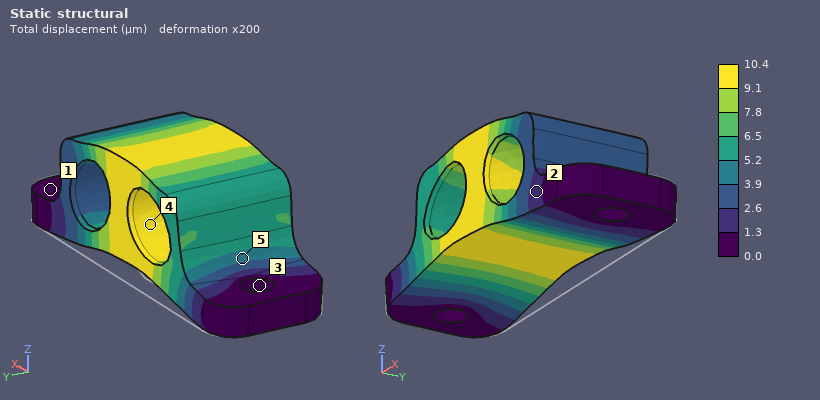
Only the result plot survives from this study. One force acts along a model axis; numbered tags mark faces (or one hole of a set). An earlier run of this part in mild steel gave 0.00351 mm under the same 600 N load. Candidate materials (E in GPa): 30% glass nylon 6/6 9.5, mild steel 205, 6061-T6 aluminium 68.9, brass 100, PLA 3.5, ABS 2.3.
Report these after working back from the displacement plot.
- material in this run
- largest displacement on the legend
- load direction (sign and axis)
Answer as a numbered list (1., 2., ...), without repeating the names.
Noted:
1. 6061-T6 aluminium
2. 10.4 µm
3. +Z
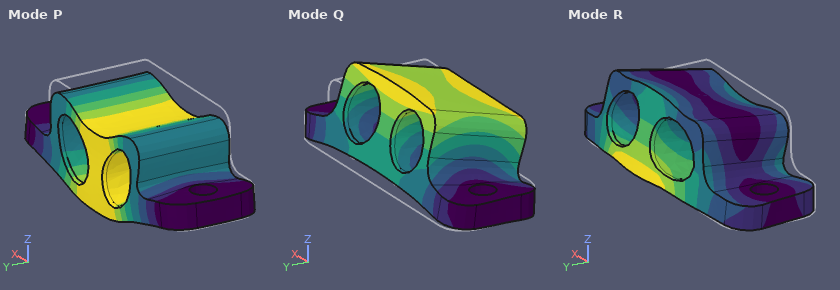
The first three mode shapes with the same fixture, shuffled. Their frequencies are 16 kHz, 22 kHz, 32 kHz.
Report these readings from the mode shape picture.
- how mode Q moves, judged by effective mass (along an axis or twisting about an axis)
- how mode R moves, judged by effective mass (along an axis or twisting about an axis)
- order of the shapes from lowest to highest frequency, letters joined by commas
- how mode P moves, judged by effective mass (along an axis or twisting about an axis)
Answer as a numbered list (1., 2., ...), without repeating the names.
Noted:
1. along Y
2. along Y
3. Q, P, R
4. along Z
